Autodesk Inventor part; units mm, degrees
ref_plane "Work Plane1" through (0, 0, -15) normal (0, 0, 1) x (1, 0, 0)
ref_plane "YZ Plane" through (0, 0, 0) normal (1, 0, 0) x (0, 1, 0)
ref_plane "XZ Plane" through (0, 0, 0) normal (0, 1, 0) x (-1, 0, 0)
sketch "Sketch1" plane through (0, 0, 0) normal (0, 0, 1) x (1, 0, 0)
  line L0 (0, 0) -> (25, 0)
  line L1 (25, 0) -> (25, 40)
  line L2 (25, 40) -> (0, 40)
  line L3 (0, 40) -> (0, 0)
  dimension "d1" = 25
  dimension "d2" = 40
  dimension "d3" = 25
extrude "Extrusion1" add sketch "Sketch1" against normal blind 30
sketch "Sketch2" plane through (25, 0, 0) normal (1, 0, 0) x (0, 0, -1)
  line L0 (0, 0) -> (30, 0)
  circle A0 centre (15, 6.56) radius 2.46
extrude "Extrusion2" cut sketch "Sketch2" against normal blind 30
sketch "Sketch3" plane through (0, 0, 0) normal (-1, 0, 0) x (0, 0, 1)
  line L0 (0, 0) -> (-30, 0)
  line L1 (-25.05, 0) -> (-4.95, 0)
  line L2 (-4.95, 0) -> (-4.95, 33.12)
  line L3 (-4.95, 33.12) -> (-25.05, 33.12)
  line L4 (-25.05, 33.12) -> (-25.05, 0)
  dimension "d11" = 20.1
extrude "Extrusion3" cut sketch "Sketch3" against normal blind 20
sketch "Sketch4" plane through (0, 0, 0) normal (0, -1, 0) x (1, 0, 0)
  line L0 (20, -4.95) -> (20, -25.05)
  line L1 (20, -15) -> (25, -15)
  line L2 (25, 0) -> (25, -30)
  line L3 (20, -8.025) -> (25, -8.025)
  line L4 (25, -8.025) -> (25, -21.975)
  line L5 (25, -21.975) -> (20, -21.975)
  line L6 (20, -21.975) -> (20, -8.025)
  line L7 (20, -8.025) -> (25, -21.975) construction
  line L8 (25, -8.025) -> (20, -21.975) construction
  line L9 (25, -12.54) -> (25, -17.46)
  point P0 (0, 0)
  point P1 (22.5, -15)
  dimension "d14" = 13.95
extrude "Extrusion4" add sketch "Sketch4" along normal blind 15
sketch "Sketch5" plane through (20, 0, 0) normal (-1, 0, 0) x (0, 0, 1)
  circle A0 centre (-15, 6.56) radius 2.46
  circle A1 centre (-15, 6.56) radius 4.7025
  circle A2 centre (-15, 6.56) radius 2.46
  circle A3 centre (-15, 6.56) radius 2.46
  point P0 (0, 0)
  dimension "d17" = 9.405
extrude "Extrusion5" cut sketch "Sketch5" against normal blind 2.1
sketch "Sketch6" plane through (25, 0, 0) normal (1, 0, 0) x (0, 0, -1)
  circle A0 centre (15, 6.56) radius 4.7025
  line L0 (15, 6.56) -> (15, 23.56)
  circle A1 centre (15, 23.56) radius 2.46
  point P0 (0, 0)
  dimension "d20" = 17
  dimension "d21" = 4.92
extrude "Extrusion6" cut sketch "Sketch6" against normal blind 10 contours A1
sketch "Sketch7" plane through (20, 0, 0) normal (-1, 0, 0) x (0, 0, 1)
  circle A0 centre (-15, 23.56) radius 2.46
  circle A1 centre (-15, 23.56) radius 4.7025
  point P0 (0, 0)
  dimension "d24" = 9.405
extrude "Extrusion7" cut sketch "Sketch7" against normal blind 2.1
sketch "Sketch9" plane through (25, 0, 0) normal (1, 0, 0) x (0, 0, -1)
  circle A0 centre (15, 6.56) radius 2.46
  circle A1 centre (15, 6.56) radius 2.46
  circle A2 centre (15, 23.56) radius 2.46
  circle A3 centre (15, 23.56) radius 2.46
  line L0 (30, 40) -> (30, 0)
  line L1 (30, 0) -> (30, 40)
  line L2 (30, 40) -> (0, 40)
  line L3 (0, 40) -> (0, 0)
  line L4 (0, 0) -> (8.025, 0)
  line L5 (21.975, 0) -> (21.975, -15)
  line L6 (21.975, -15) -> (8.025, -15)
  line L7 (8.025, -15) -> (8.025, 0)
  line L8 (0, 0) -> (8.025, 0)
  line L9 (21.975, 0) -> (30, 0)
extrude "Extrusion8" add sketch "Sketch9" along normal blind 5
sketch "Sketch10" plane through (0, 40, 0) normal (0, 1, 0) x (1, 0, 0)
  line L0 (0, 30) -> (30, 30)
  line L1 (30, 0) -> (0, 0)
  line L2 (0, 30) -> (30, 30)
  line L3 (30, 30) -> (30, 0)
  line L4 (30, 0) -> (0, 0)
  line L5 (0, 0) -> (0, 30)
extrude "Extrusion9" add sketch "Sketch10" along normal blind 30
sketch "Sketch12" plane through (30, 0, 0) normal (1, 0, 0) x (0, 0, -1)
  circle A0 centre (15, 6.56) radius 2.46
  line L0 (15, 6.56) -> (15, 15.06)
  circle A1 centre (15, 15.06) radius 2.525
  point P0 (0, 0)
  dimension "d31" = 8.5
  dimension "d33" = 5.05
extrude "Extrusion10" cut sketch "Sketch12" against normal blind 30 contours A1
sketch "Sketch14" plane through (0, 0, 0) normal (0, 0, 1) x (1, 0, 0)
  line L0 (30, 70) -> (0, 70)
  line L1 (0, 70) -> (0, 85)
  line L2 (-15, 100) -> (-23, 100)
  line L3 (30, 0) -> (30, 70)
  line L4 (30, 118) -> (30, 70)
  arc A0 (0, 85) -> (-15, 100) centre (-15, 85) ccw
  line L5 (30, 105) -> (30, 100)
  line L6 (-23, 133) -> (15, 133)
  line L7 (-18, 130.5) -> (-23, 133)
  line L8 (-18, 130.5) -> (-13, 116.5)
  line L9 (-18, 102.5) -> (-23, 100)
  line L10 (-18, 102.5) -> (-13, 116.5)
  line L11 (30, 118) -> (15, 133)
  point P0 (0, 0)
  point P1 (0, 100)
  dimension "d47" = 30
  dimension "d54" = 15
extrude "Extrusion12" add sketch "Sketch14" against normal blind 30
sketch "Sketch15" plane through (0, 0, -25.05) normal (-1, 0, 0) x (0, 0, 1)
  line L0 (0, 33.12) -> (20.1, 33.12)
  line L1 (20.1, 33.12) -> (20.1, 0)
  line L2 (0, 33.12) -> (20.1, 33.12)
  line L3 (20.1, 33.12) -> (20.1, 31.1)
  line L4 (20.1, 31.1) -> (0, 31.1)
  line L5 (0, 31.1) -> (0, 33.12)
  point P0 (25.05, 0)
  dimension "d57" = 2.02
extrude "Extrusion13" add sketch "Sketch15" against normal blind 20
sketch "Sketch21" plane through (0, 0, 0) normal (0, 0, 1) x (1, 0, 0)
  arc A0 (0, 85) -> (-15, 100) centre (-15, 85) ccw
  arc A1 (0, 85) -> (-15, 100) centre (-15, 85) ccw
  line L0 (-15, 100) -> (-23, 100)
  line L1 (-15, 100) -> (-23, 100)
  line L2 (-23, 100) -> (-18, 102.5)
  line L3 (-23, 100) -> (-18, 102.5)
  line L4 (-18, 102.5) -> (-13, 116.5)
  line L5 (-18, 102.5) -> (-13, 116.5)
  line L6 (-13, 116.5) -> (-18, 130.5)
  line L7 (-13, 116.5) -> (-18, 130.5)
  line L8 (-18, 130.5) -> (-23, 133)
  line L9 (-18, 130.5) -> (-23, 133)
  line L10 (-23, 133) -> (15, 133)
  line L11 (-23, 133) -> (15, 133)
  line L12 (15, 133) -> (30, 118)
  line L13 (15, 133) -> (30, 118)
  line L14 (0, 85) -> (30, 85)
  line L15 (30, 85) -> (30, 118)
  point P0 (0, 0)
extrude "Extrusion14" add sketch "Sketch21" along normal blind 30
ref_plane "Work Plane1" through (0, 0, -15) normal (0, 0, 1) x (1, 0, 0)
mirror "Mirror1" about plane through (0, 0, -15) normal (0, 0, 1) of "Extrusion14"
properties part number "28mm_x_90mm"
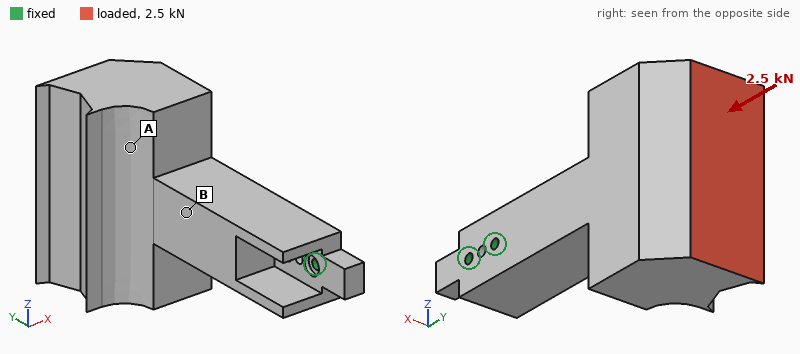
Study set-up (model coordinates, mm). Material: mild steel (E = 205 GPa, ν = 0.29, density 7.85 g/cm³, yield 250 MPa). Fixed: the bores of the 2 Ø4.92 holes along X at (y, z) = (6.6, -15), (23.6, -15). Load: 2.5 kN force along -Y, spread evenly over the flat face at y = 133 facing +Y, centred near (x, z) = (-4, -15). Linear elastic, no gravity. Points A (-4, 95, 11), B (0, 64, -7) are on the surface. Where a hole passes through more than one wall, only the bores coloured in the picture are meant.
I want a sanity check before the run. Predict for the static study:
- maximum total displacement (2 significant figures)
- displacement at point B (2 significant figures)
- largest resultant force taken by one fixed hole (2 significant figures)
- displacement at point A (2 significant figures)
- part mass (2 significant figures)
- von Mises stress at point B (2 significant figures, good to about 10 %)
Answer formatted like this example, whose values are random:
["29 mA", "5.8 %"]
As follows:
["84 µm", "29 µm", "3.4 kN", "50 µm", "1.9 kg", "13 MPa"]
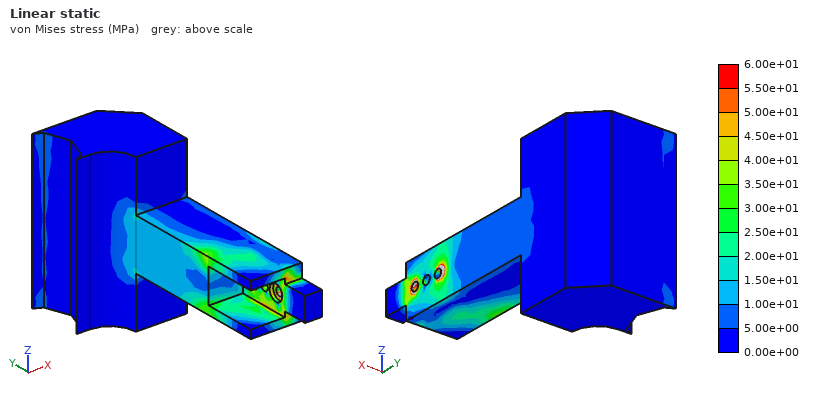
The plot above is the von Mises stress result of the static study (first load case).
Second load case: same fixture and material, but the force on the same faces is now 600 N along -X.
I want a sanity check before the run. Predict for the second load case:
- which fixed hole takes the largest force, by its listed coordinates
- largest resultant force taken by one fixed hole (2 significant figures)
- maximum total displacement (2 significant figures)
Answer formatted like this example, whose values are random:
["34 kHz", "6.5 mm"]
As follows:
["(23.6, -15)", "3.2 kN", "76 µm"]
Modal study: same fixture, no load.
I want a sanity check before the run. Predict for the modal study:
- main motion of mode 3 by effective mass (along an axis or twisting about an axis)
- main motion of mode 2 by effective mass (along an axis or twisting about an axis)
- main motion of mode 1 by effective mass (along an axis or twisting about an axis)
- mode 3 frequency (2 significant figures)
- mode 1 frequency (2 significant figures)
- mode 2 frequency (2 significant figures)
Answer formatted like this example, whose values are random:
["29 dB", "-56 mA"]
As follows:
["twisting about Y", "along Z", "along X", "990 Hz", "490 Hz", "550 Hz"]
